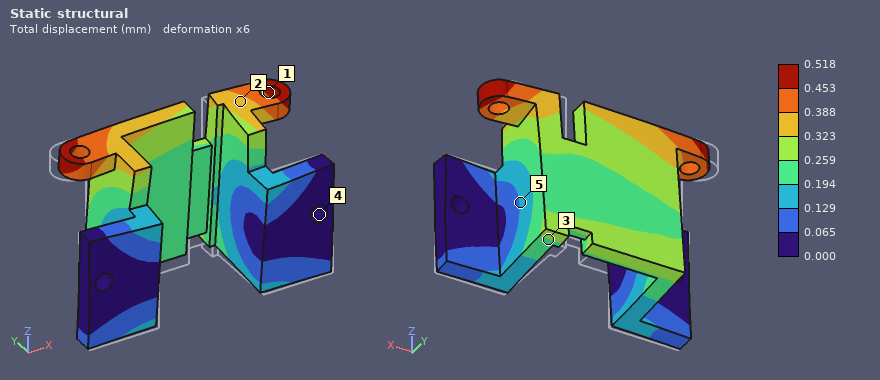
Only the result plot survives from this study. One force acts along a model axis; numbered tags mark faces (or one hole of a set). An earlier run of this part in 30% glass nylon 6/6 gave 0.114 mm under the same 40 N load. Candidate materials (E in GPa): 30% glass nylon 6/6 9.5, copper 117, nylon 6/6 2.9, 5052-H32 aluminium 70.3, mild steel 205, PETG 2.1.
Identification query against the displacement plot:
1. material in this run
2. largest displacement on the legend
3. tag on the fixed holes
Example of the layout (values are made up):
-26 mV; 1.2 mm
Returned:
PETG; 0.518 mm; 4
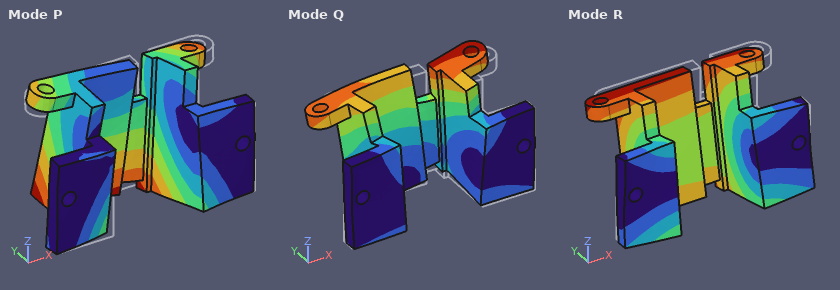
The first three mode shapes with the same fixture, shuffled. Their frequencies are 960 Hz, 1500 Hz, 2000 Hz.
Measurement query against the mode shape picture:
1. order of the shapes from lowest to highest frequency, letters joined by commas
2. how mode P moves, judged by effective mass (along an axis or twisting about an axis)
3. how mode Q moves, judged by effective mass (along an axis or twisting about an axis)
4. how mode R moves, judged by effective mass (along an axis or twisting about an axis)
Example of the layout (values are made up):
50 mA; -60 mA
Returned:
R, Q, P; along X; along X; along Z
